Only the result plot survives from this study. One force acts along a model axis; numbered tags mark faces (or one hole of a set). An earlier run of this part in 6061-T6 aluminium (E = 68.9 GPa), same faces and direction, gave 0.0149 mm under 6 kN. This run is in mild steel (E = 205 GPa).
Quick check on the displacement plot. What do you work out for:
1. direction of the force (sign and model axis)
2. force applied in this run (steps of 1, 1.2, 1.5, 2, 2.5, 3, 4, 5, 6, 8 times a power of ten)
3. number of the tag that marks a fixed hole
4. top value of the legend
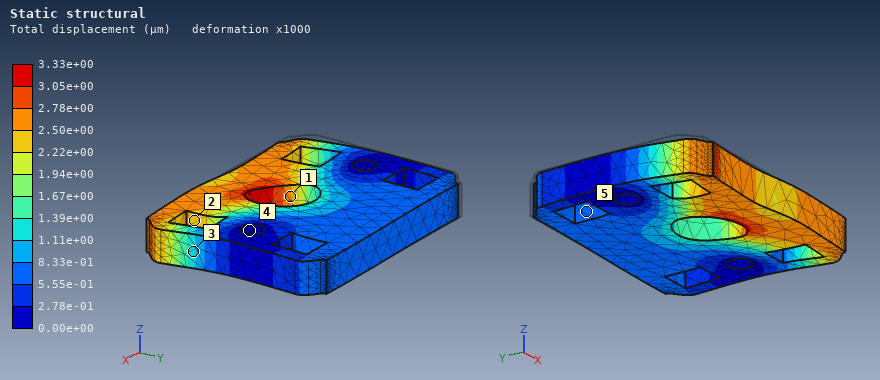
+X
4 kN
4
3.33e+00 µm
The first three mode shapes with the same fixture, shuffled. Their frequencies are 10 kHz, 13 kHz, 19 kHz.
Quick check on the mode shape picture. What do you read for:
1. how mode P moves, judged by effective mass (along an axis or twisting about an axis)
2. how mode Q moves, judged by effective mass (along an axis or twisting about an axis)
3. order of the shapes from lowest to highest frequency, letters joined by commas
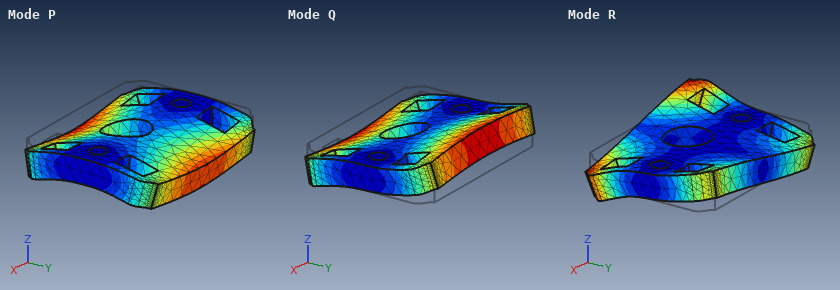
along Z
twisting about X
Q, P, R
